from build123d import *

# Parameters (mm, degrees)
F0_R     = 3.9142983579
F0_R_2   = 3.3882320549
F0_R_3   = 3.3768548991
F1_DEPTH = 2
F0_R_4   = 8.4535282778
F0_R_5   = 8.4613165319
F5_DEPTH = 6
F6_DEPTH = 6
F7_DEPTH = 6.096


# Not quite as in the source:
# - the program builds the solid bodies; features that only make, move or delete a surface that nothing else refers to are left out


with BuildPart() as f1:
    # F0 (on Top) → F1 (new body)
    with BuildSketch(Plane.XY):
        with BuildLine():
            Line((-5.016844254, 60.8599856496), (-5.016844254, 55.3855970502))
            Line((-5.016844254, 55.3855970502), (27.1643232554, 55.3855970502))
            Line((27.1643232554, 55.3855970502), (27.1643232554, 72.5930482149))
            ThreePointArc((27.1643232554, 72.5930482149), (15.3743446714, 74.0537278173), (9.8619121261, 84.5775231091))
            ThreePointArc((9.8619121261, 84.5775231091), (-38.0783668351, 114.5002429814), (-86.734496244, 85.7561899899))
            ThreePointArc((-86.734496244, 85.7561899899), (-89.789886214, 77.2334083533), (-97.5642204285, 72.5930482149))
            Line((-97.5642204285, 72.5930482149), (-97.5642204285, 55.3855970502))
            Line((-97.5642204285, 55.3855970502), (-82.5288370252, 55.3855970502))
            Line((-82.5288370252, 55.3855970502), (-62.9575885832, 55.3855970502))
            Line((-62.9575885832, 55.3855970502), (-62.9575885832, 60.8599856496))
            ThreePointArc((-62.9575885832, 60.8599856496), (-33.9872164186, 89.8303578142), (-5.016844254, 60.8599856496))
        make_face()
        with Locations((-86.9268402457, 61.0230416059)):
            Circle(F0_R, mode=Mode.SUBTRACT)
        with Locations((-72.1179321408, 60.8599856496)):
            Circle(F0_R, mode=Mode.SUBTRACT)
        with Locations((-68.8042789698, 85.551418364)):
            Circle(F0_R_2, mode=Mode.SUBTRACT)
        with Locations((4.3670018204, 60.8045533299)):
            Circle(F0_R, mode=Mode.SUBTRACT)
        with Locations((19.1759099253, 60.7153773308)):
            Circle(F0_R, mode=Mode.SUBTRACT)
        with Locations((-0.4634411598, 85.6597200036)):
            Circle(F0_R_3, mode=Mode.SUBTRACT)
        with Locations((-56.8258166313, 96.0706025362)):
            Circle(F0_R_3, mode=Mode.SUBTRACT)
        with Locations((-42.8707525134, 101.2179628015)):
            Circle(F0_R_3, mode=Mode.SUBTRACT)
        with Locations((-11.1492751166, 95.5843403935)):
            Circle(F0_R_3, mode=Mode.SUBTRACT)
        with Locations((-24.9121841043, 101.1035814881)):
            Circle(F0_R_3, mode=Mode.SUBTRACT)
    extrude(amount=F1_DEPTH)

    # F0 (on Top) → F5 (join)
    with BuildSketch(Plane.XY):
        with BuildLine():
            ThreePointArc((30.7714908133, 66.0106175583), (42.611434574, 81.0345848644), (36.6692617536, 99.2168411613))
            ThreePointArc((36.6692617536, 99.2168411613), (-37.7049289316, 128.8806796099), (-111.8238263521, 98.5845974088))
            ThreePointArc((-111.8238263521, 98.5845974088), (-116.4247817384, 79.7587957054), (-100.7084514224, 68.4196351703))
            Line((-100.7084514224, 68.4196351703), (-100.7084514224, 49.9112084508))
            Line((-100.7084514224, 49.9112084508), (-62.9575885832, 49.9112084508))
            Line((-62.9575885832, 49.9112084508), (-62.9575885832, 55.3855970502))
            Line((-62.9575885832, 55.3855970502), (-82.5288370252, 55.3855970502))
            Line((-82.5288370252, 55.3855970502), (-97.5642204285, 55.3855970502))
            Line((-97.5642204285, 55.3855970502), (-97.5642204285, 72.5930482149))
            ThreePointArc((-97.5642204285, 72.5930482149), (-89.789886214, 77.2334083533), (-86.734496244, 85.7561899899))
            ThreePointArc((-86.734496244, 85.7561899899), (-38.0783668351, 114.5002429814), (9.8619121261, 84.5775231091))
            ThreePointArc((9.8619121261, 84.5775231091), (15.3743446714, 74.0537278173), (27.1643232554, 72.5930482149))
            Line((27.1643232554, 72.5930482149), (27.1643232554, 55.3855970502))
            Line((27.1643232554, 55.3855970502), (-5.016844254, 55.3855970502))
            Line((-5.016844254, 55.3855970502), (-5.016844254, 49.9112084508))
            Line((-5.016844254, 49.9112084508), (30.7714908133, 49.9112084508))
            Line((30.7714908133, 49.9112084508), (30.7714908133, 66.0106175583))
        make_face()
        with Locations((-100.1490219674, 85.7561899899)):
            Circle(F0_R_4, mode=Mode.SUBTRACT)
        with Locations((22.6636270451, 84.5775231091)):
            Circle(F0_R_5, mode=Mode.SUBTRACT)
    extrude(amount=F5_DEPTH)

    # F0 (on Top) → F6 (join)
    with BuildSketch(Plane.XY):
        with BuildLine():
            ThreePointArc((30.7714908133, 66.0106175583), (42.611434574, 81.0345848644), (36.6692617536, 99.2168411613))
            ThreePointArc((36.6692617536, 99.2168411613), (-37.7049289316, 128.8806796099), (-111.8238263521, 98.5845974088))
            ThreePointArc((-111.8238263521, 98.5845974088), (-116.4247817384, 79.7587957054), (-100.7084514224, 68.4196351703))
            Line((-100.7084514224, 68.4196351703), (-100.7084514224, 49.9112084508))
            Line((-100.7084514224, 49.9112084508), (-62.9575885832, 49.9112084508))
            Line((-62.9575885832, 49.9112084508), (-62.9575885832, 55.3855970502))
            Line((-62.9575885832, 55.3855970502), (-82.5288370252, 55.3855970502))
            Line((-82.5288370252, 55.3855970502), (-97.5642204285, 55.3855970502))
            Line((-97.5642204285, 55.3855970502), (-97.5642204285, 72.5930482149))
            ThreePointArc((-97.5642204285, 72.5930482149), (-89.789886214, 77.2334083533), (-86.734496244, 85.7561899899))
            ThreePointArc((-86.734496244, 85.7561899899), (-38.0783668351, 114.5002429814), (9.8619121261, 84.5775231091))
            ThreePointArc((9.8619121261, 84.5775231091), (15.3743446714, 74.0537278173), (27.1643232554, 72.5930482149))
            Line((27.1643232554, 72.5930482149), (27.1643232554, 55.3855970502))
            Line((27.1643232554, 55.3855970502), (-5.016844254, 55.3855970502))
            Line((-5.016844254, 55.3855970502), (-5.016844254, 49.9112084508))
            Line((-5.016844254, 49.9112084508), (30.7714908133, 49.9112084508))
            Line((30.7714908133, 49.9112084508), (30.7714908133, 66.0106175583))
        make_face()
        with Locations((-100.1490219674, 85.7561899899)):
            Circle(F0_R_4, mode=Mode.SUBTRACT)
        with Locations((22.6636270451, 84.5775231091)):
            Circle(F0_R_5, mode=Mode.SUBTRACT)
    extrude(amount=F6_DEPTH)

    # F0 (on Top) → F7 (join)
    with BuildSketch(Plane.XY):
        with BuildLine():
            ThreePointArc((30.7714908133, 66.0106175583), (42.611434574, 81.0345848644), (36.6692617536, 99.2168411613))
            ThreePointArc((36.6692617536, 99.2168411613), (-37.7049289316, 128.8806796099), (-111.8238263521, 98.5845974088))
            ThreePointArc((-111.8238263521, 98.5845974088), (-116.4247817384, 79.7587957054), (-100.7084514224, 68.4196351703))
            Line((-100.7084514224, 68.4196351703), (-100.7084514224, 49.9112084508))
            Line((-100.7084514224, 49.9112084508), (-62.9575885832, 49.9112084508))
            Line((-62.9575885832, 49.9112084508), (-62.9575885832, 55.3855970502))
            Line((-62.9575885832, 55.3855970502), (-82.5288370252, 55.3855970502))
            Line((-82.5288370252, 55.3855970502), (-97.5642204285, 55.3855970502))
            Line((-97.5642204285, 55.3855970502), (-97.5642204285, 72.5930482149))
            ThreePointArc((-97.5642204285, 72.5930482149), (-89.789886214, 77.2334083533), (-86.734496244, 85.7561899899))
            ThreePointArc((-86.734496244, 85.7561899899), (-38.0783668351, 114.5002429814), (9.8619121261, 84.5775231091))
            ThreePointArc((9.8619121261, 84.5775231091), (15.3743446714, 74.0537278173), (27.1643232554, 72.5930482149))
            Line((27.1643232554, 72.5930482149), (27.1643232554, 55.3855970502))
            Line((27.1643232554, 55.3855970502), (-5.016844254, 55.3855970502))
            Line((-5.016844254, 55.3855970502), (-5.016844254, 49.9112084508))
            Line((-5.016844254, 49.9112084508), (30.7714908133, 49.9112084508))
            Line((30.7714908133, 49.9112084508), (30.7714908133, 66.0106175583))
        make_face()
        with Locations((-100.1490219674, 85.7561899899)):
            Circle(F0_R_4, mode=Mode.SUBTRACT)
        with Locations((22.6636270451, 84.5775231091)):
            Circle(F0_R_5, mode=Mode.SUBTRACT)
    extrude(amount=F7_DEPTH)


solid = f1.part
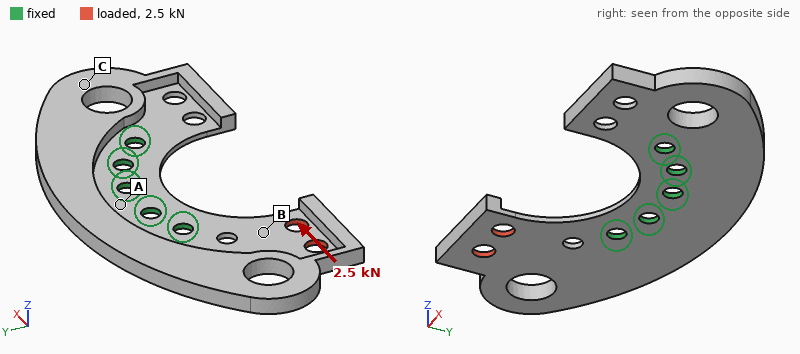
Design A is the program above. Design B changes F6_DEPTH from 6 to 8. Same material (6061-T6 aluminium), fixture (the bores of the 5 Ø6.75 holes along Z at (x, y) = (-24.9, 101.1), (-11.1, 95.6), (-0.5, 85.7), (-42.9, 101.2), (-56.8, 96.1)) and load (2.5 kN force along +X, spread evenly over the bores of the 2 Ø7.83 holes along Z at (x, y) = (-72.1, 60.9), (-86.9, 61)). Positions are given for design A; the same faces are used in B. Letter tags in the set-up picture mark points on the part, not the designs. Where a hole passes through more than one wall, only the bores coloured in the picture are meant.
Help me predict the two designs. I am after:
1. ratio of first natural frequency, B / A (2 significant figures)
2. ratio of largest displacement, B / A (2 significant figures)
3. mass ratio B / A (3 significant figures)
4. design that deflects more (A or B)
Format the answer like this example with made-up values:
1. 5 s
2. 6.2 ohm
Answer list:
1. 1.1
2. 0.82
3. 1.24
4. A
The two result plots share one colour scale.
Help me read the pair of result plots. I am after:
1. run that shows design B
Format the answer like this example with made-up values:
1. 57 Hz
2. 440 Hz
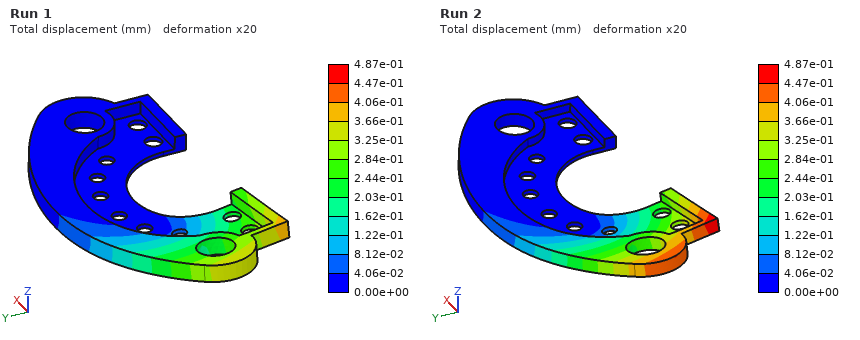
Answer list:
1. Run 1
